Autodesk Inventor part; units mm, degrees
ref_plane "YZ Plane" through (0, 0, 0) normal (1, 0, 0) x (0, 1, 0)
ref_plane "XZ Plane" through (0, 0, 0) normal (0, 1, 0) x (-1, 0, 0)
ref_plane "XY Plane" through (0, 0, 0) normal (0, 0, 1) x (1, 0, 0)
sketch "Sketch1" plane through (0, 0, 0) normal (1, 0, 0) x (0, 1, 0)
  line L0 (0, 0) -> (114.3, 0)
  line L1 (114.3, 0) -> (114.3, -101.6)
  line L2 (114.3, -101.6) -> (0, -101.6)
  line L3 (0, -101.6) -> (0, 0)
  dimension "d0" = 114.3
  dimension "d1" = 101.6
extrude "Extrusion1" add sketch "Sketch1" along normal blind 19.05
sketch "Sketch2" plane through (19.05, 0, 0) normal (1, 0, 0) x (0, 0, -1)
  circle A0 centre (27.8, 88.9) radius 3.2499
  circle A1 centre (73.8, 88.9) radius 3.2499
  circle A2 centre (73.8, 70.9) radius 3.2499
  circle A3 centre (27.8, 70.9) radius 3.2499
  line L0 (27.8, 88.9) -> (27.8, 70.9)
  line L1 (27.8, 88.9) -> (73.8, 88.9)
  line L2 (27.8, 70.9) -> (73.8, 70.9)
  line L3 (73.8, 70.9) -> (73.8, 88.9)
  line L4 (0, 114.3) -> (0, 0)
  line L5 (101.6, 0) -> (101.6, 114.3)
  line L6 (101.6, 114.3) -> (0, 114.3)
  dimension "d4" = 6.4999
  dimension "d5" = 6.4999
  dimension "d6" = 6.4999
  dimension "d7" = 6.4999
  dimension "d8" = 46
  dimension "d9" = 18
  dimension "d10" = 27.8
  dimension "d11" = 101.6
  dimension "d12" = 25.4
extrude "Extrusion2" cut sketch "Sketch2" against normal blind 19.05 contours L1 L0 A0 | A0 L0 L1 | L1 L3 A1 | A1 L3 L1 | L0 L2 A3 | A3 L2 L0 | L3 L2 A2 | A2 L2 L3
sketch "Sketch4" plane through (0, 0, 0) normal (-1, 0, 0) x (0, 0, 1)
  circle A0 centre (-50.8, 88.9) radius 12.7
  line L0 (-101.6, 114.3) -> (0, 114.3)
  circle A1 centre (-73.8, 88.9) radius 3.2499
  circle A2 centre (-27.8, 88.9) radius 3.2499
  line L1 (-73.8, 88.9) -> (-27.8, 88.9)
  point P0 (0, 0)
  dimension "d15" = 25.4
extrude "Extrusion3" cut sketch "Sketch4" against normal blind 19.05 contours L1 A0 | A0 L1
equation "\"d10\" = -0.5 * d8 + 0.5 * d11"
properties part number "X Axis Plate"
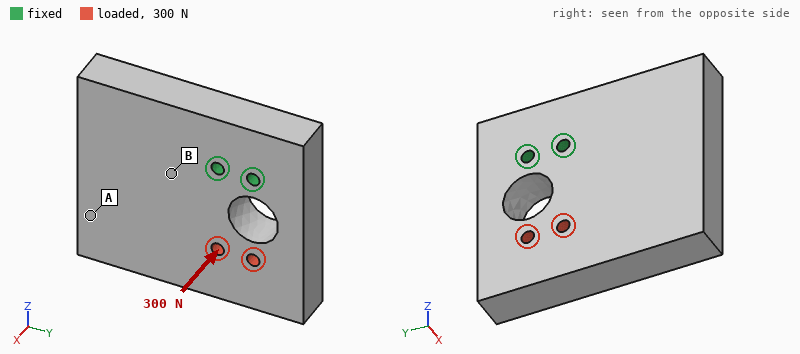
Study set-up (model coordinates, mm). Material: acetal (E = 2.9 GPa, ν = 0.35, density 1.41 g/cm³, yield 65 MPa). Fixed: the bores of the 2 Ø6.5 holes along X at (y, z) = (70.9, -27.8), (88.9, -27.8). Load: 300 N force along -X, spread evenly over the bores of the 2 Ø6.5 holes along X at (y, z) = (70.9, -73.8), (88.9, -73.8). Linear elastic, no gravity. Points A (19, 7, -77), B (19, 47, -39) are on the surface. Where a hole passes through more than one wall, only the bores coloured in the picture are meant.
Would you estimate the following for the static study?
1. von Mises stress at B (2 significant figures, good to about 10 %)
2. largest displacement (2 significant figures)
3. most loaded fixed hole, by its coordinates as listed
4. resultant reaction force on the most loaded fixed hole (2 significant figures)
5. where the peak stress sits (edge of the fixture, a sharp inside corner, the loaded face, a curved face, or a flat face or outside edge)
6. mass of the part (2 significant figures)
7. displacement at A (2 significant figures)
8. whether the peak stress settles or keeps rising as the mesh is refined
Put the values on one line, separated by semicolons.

1.3 MPa; 0.27 mm; (70.9, -27.8); 170 N; edge of the fixture; 290 g; 0.12 mm; keeps rising
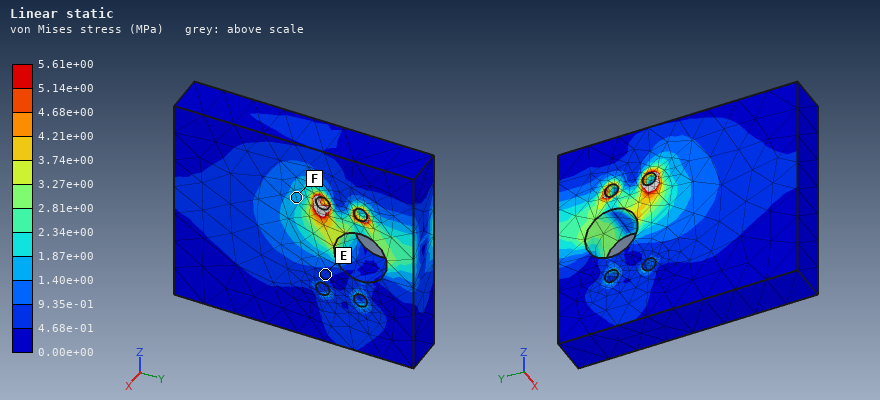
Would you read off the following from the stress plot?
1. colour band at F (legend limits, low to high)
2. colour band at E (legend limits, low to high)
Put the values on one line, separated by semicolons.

1.40e+00 to 1.87e+00 MPa; 4.68e-01 to 9.35e-01 MPa
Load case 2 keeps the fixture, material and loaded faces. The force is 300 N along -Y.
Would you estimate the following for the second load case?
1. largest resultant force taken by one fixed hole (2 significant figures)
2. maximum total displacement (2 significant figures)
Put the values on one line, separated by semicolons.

580 N; 0.12 mm
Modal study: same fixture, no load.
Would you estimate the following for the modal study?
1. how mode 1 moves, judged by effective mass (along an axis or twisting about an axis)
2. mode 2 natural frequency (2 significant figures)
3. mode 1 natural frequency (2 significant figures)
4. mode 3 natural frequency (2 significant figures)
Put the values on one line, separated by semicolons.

along X; 610 Hz; 450 Hz; 660 Hz
